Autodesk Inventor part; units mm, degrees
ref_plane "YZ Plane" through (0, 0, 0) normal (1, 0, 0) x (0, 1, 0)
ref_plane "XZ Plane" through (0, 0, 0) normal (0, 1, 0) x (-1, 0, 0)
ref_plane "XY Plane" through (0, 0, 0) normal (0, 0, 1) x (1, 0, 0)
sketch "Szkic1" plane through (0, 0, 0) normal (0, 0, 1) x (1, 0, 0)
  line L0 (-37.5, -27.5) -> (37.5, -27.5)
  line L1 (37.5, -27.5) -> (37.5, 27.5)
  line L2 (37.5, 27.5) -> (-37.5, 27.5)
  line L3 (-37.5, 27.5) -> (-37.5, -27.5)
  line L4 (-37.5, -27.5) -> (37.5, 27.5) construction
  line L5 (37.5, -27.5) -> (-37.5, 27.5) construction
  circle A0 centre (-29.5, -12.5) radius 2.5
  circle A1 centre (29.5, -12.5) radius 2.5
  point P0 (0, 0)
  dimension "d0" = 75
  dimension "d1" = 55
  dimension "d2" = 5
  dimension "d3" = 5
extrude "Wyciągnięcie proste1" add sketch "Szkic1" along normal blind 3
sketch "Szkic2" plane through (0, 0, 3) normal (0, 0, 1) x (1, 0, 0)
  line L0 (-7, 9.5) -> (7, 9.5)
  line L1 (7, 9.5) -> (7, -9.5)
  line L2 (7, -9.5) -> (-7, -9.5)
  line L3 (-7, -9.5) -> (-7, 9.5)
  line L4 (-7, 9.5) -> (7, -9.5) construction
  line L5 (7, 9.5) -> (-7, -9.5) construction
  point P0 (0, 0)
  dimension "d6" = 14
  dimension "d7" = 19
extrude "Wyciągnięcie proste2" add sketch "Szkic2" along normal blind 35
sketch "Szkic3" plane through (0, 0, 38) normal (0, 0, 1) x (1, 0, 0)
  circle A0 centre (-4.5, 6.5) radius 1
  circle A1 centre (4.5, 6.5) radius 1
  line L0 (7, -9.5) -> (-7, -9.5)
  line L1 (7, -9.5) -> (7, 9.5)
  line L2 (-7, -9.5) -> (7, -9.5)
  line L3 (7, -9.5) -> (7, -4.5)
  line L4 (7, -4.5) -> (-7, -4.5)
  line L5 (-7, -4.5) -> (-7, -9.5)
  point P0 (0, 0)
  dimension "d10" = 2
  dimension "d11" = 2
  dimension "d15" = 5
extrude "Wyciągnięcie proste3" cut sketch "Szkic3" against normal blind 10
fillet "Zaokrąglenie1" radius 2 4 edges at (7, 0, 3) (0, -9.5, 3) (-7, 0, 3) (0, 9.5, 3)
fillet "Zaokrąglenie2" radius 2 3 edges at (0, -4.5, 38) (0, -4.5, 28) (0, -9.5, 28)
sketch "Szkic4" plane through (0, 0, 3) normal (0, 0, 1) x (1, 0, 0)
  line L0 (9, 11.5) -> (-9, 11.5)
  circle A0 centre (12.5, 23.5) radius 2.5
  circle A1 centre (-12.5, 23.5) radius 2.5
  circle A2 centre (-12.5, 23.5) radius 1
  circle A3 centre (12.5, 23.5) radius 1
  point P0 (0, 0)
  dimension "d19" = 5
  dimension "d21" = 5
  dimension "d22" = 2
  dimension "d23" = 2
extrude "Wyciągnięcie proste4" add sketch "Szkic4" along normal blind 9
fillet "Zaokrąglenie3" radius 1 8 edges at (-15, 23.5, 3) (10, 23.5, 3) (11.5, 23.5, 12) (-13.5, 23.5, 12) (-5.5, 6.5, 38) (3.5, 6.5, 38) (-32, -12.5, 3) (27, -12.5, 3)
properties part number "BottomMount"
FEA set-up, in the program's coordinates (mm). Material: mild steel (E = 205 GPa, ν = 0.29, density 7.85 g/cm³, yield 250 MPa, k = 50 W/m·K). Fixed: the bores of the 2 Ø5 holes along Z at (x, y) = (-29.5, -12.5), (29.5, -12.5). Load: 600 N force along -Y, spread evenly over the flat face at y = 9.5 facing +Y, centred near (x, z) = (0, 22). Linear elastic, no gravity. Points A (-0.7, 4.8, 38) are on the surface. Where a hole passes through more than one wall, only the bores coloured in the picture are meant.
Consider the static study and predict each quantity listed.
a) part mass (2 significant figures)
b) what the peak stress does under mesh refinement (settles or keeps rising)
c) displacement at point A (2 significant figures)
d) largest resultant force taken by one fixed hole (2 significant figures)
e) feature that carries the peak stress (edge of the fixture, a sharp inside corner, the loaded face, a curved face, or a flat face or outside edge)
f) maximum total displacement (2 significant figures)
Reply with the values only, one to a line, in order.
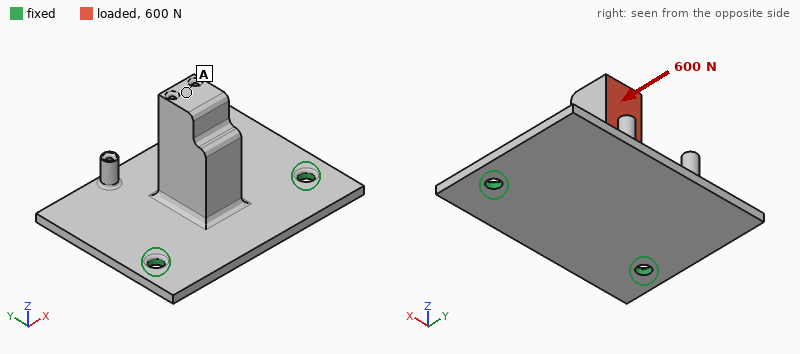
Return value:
170 g
keeps rising
0.23 mm
310 N
edge of the fixture
0.24 mm
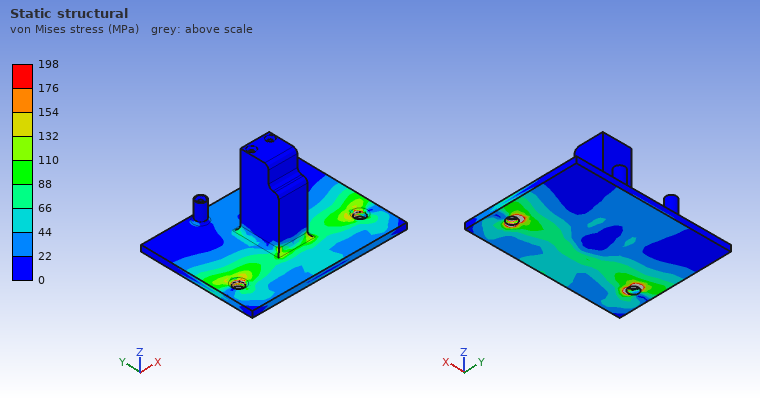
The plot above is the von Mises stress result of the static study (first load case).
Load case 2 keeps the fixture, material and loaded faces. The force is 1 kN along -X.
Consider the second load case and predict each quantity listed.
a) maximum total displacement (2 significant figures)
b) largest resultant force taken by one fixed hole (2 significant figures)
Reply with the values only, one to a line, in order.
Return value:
97 µm
760 N
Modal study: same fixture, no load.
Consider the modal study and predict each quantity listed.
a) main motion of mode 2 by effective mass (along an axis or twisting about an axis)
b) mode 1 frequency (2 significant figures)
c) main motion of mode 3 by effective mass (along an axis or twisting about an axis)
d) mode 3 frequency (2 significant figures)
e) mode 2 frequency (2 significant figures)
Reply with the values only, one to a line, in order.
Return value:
along X
890 Hz
along Z
2500 Hz
2300 Hz
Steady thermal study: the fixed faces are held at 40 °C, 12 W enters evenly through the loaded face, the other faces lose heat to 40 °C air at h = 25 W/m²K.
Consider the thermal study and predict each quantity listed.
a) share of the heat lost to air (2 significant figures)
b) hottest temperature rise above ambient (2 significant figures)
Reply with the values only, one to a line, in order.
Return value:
39 %
42 K
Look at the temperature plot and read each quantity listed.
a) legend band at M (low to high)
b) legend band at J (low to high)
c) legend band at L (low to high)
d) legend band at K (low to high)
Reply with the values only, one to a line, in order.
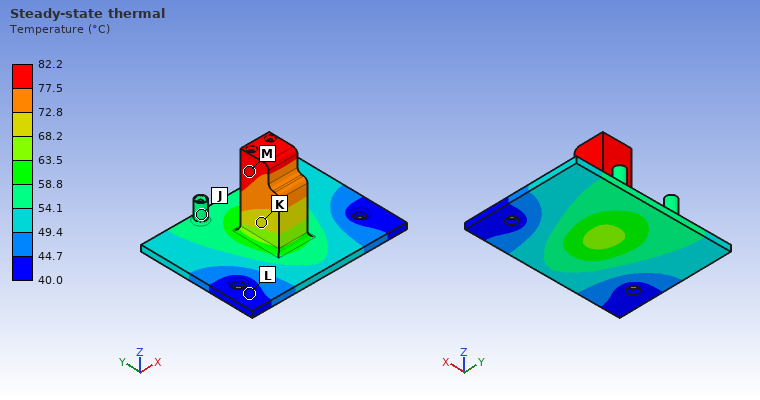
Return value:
77.5 to 82.2 °C
54.1 to 58.8 °C
40.0 to 44.7 °C
68.2 to 72.8 °C
